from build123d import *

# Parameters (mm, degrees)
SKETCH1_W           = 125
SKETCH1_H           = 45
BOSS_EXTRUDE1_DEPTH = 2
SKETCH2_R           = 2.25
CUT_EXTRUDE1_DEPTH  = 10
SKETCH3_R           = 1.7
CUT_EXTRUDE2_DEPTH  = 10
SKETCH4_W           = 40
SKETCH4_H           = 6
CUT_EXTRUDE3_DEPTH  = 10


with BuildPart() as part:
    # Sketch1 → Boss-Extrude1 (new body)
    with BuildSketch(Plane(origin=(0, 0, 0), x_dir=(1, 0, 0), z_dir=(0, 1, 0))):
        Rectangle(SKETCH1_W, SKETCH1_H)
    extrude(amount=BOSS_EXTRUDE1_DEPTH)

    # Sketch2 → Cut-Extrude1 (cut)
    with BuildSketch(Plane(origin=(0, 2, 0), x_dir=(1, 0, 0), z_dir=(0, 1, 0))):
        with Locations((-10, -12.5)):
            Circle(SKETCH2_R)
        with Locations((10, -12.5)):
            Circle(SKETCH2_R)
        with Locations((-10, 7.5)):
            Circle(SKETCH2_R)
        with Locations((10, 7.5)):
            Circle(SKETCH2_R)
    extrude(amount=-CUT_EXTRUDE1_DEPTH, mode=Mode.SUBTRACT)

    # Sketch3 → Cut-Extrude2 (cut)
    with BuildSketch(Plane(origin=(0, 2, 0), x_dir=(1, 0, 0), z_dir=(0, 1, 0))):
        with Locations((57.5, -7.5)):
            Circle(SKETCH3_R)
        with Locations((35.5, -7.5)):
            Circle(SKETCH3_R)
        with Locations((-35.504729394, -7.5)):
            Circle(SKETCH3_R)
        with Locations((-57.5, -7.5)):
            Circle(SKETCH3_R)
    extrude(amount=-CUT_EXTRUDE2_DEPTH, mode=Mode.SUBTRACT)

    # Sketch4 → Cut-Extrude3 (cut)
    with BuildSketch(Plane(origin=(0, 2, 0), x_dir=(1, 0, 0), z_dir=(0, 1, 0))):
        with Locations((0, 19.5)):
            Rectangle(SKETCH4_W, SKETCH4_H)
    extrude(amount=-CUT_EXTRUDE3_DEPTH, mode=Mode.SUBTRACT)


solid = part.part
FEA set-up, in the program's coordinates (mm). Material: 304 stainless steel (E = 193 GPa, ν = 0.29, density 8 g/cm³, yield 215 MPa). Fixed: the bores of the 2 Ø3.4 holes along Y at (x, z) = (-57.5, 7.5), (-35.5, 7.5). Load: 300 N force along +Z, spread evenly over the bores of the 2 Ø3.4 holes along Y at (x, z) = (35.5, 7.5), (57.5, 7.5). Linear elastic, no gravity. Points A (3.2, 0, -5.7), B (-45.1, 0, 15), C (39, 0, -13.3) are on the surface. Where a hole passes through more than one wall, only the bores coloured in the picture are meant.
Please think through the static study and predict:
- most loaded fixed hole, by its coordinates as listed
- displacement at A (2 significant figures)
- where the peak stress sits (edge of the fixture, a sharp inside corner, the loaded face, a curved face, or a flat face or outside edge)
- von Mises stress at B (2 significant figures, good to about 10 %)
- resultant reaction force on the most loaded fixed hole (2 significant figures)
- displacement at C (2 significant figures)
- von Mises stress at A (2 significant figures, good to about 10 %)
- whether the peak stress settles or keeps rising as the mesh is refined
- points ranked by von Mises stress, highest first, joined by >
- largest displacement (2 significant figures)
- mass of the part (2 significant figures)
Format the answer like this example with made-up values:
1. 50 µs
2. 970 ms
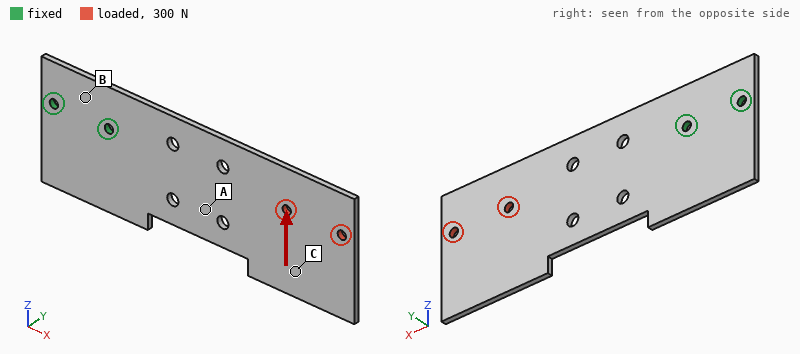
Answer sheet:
1. (-35.5, 7.5)
2. 25 µm
3. edge of the fixture
4. 25 MPa
5. 1.3 kN
6. 57 µm
7. 15 MPa
8. keeps rising
9. B > A > C
10. 79 µm
11. 85 g
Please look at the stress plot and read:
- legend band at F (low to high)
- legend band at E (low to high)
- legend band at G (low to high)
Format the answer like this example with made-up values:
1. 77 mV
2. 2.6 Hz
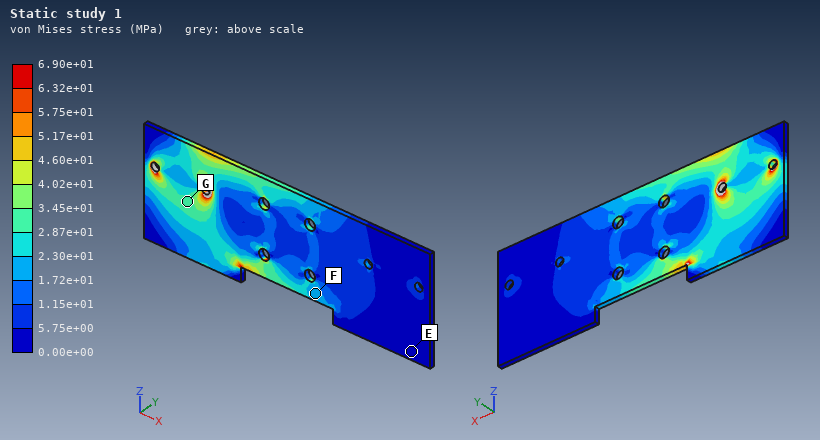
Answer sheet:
1. 1.72e+01 to 2.30e+01 MPa
2. 0.00e+00 to 5.75e+00 MPa
3. 2.87e+01 to 3.45e+01 MPa
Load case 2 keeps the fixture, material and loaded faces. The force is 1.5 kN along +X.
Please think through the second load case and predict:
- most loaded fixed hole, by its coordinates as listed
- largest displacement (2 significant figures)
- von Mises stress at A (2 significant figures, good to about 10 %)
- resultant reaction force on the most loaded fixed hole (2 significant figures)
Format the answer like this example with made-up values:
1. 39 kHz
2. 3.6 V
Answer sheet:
1. (-35.5, 7.5)
2. 21 µm
3. 12 MPa
4. 1.1 kN
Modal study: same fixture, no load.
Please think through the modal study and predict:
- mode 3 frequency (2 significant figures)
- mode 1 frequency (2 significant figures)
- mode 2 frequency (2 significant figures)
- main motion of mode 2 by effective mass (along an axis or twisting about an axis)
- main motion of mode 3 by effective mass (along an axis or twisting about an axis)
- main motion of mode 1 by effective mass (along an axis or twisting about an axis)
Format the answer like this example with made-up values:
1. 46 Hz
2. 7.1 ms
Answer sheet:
1. 980 Hz
2. 150 Hz
3. 650 Hz
4. twisting about X
5. along Y
6. along Y
